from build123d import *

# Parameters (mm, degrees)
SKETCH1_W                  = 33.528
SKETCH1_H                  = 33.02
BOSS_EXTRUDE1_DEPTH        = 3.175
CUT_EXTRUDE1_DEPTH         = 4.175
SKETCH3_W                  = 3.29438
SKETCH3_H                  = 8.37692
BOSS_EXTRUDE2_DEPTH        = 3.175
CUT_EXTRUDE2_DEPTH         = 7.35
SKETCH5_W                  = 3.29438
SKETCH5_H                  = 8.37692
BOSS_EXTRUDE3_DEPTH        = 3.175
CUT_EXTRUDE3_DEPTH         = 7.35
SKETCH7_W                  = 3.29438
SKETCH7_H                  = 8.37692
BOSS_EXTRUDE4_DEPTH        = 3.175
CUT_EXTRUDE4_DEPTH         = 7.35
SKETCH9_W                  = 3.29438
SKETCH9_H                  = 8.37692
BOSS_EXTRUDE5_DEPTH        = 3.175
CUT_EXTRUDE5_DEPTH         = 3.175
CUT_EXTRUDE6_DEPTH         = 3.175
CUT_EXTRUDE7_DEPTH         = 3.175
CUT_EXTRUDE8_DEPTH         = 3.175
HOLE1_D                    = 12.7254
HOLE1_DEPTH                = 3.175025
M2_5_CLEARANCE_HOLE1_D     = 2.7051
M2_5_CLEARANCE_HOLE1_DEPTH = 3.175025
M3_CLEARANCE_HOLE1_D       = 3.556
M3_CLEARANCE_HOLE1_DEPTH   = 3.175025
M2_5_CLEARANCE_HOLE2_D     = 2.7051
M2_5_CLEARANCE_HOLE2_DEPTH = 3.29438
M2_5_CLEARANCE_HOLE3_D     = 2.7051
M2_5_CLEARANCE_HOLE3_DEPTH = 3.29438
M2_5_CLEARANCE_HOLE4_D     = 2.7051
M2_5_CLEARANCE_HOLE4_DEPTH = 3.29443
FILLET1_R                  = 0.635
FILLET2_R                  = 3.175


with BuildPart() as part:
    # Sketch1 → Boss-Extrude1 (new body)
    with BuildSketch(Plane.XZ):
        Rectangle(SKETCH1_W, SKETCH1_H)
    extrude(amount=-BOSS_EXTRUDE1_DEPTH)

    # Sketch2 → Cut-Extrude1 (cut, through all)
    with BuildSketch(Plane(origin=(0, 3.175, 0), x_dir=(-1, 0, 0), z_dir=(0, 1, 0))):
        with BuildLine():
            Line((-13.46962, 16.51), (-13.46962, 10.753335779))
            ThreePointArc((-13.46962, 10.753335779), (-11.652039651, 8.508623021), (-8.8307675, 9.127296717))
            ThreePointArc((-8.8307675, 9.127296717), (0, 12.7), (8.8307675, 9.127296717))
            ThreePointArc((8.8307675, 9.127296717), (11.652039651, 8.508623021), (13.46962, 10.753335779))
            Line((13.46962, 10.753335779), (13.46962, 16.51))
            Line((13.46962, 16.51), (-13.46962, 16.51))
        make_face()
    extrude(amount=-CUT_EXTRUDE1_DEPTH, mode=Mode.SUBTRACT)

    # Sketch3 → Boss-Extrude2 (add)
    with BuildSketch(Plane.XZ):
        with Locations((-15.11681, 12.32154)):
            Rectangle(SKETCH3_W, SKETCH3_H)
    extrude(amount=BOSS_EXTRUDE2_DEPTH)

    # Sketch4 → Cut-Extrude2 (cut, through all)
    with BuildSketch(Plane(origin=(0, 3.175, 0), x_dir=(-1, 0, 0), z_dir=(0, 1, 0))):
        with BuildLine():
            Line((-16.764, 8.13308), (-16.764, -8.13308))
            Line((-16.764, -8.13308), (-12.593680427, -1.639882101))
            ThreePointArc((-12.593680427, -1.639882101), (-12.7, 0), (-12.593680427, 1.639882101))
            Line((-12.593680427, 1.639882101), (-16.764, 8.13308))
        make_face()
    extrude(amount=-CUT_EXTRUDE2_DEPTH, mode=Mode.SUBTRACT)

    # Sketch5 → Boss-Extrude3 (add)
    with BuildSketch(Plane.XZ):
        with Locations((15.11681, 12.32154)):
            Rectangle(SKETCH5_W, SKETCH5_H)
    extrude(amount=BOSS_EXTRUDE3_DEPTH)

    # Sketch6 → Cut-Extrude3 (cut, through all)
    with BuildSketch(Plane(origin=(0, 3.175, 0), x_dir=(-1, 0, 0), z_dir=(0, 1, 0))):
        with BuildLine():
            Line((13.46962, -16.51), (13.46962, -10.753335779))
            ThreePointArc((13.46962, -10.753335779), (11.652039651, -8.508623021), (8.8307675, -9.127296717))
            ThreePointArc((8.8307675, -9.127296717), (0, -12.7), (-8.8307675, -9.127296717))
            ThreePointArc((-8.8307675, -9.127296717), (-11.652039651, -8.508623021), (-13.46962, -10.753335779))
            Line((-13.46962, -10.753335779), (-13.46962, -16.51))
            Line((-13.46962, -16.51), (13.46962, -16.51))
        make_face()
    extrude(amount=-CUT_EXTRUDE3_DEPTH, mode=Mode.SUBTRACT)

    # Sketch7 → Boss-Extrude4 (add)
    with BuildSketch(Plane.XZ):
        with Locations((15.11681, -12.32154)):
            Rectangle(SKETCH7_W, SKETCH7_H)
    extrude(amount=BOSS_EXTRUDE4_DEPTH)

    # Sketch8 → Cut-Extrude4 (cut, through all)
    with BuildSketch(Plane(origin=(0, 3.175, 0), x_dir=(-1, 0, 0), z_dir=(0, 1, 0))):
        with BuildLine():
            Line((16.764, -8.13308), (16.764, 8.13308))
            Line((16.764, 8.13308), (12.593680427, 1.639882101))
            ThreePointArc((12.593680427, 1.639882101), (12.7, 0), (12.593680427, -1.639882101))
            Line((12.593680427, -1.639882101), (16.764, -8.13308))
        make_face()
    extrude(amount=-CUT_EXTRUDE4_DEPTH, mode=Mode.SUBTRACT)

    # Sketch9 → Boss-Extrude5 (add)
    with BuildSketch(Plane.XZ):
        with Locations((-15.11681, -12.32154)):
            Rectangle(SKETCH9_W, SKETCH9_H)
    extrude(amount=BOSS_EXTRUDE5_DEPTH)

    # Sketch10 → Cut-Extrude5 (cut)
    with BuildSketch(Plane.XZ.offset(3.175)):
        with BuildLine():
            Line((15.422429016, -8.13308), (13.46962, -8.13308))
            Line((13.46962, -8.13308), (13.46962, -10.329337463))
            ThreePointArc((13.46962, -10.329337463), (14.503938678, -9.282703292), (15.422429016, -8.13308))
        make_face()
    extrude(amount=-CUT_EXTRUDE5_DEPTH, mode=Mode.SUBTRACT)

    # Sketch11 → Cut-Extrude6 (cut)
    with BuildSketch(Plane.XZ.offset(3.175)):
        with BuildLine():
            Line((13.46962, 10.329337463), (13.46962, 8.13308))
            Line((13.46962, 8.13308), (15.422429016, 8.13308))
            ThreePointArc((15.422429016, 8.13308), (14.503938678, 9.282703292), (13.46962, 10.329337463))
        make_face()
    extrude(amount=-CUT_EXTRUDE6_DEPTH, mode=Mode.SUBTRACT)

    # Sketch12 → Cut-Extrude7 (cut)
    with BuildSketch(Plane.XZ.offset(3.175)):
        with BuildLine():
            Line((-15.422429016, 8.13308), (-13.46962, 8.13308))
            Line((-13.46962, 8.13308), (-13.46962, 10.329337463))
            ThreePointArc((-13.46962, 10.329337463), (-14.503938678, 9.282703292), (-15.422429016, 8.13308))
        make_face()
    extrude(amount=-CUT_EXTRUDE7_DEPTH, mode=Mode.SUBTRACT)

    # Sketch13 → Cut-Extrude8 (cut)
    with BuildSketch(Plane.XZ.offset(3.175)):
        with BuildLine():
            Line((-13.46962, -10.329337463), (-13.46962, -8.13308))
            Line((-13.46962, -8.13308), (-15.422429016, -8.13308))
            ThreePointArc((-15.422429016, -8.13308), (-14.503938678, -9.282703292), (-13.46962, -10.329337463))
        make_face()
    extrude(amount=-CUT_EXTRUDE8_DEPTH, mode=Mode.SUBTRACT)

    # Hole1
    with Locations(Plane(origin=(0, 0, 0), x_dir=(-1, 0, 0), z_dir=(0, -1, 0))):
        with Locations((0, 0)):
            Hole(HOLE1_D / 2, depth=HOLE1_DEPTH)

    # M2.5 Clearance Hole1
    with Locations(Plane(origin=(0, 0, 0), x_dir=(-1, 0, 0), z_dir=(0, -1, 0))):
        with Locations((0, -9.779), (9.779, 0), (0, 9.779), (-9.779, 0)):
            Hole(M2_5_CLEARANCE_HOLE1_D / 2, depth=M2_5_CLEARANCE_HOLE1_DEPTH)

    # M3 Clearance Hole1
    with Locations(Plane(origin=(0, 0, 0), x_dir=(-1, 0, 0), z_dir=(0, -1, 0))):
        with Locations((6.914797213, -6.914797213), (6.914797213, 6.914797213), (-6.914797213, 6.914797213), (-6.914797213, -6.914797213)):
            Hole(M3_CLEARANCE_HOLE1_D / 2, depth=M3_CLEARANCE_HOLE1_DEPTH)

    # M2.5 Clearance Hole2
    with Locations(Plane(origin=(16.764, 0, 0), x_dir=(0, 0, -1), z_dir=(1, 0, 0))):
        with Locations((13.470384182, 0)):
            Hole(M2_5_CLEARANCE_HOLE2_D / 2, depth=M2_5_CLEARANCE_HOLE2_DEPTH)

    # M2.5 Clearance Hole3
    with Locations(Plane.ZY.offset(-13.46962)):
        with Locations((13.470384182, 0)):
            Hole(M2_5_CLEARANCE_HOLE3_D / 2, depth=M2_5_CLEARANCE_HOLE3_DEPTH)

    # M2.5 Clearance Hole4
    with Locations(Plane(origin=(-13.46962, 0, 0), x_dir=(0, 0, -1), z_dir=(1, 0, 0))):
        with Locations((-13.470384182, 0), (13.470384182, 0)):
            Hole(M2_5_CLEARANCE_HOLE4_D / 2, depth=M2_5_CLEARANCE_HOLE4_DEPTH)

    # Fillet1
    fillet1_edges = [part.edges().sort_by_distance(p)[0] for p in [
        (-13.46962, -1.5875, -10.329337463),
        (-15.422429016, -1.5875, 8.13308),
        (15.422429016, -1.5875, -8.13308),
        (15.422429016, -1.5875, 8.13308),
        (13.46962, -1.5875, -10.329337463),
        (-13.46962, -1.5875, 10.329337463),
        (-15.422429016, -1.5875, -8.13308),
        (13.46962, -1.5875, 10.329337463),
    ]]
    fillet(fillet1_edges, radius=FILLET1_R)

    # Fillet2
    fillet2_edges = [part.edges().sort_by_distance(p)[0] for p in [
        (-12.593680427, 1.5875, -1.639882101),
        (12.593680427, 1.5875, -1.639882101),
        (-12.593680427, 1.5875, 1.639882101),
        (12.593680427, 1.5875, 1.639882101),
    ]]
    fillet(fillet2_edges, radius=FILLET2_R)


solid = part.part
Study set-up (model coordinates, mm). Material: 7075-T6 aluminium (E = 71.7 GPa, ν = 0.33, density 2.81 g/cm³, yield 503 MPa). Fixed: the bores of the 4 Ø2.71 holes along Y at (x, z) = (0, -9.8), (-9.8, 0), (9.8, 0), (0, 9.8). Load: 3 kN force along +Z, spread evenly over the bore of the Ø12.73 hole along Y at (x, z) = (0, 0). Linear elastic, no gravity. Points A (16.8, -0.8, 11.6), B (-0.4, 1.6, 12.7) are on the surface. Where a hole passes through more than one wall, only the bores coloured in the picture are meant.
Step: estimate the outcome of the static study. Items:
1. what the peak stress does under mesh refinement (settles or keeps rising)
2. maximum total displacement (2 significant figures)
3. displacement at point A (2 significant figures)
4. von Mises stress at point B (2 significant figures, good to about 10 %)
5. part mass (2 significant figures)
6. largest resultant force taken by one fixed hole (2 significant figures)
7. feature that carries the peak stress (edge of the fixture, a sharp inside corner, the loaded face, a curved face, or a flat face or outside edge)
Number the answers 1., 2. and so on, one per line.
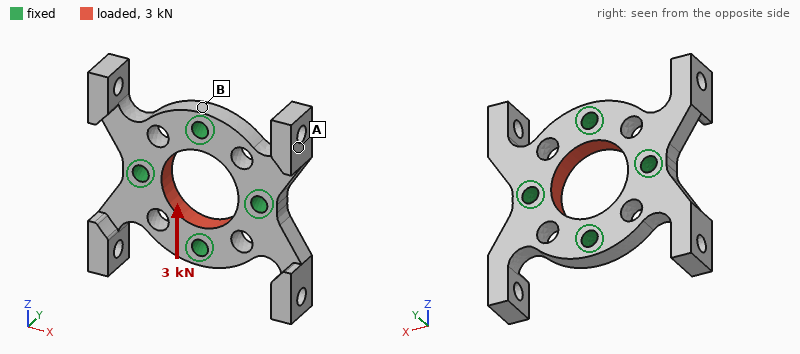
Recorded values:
1. keeps rising
2. 4.7 µm
3. 3.1 µm
4. 21 MPa
5. 5.3 g
6. 770 N
7. edge of the fixture
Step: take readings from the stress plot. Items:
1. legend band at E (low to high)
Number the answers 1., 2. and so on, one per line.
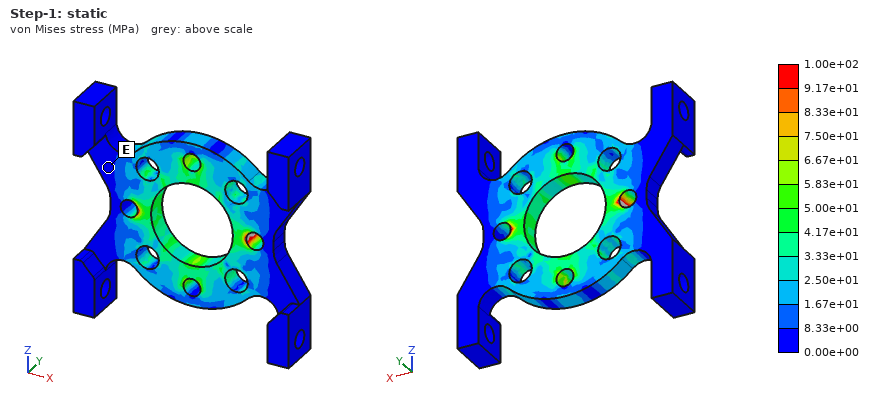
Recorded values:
1. 0.00e+00 to 8.33e+00 MPa
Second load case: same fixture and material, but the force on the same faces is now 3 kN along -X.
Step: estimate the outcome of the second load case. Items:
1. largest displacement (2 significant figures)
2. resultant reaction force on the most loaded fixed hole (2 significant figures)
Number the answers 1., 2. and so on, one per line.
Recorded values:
1. 4.8 µm
2. 750 N
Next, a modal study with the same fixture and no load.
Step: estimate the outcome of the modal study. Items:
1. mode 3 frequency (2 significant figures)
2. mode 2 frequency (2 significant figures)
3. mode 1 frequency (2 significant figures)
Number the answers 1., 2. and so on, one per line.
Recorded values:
1. 9200 Hz
2. 9200 Hz
3. 9100 Hz
